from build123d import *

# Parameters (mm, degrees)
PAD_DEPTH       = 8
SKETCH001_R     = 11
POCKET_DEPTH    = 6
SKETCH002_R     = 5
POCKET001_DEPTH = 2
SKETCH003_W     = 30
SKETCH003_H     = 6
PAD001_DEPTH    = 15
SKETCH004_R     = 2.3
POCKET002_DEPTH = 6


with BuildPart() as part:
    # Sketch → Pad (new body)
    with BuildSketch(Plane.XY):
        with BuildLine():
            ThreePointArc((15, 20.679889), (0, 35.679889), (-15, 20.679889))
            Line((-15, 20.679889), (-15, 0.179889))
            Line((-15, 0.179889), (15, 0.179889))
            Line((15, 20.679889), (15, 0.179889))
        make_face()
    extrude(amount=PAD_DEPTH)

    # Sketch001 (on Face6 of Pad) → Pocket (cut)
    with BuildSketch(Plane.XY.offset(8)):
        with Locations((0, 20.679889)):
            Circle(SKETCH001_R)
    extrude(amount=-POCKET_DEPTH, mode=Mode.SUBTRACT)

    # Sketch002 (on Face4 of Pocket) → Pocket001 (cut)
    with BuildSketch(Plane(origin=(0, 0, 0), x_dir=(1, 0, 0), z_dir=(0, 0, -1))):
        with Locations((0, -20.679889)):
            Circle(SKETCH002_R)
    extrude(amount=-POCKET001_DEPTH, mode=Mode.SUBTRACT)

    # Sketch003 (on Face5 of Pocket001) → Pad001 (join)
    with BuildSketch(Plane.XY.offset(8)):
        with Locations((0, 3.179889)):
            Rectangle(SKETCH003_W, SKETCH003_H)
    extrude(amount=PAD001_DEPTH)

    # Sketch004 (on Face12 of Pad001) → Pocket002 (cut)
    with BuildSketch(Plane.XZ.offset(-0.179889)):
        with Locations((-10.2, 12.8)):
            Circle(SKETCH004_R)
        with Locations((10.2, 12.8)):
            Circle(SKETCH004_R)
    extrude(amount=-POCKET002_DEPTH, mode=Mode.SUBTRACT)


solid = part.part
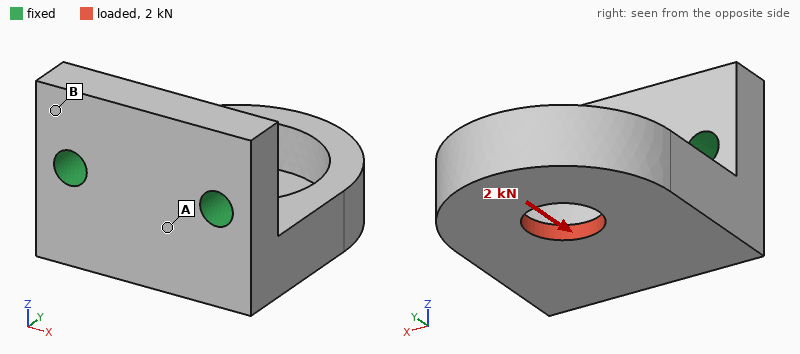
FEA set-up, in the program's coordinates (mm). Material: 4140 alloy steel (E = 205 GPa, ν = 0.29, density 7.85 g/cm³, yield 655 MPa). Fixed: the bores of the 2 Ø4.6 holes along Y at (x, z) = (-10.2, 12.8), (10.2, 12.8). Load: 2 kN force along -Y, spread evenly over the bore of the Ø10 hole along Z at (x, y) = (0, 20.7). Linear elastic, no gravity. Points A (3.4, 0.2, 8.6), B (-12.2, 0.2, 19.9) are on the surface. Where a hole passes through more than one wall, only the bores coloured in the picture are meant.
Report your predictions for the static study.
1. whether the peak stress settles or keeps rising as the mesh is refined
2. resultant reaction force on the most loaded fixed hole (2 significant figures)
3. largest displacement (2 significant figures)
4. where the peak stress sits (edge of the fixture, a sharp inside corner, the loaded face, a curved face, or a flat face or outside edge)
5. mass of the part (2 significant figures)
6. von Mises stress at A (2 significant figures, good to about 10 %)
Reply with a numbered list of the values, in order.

1. keeps rising
2. 1.0 kN
3. 46 µm
4. edge of the fixture
5. 61 g
6. 50 MPa
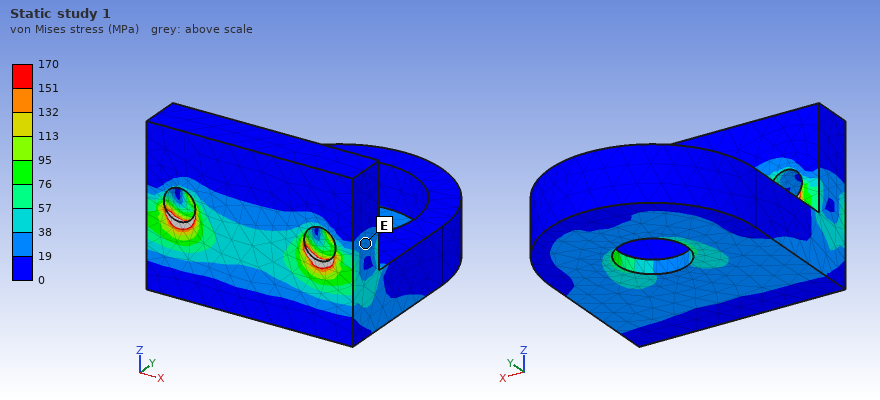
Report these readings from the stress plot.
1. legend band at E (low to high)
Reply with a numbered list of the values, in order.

1. 19 to 38 MPa
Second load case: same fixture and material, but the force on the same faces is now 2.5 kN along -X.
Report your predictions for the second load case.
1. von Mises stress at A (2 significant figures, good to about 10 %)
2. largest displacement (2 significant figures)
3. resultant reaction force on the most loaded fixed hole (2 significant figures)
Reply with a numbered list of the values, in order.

1. 18 MPa
2. 32 µm
3. 2.5 kN
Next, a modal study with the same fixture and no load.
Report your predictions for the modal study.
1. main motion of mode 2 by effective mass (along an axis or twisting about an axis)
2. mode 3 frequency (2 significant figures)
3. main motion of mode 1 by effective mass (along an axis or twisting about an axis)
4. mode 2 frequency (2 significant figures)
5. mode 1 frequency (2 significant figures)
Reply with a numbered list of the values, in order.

1. along X
2. 15 kHz
3. along Z
4. 8600 Hz
5. 4600 Hz
